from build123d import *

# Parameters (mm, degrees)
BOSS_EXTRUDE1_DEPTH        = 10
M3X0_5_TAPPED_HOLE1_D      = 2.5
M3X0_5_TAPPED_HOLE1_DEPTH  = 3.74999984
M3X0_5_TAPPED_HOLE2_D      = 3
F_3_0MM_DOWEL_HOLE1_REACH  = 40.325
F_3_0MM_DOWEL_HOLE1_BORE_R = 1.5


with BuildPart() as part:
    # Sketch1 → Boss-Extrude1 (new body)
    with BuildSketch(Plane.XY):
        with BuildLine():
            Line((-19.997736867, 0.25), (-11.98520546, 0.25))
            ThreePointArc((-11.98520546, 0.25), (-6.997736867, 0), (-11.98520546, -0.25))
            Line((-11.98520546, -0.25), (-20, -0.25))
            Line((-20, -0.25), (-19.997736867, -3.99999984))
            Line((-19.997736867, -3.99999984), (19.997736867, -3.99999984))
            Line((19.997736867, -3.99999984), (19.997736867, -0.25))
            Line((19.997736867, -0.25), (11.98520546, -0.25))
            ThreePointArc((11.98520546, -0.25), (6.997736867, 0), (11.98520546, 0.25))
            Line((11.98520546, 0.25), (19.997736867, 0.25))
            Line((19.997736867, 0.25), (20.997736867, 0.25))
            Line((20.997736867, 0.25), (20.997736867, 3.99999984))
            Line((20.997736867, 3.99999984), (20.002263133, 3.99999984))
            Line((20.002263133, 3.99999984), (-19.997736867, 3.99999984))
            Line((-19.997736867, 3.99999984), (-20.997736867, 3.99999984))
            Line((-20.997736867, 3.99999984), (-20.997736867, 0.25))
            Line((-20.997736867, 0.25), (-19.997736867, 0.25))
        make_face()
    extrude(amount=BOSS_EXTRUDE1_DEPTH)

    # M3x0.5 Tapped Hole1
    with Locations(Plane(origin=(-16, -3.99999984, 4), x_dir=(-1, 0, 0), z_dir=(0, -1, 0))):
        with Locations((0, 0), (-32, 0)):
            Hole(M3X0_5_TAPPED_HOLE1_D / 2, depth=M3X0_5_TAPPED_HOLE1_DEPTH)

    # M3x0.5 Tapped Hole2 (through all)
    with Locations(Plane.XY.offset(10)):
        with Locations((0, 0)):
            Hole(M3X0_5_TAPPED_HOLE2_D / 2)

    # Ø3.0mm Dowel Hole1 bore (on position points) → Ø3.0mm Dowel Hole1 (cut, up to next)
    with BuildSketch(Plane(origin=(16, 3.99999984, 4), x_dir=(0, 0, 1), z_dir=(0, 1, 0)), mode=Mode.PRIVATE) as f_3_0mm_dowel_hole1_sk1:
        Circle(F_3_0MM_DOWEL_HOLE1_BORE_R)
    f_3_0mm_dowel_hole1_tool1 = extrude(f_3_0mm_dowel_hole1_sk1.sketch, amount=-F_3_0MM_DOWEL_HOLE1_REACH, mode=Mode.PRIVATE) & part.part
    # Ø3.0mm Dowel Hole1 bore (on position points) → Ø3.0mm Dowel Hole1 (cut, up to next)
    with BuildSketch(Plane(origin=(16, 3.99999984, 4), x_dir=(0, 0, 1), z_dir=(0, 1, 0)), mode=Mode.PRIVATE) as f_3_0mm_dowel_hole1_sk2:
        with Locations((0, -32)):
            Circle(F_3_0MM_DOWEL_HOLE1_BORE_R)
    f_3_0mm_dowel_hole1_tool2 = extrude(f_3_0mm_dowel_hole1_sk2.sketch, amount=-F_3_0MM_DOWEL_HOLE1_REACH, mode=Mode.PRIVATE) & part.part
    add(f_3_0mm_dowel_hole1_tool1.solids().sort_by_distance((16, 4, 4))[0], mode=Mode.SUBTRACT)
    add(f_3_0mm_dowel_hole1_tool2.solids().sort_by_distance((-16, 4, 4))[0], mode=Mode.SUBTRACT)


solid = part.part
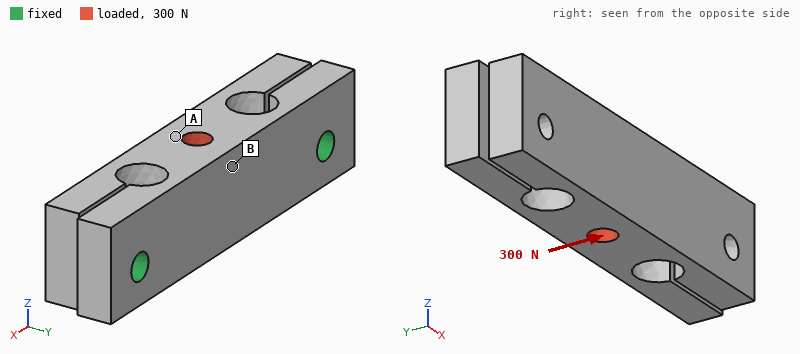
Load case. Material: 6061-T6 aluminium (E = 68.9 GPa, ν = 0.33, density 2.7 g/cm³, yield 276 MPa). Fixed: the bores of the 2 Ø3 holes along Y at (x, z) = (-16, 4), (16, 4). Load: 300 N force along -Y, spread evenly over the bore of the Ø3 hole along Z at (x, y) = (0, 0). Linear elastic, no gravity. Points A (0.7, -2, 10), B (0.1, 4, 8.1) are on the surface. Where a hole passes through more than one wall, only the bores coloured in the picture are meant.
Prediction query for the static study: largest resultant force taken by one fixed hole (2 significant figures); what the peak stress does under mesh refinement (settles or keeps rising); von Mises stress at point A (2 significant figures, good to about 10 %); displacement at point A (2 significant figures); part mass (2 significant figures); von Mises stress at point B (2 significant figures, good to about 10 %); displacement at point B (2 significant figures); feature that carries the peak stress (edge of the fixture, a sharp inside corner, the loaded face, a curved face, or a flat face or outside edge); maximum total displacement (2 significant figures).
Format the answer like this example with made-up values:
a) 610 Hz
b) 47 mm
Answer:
a) 150 N
b) keeps rising
c) 7.1 MPa
d) 14 µm
e) 7.1 g
f) 15 MPa
g) 13 µm
h) edge of the fixture
i) 14 µm
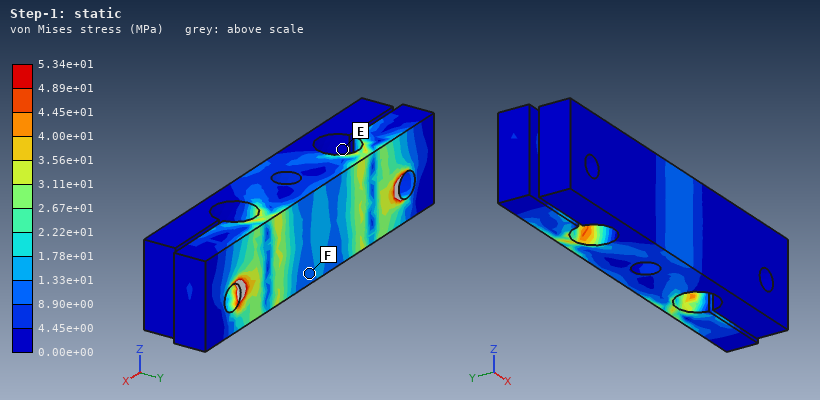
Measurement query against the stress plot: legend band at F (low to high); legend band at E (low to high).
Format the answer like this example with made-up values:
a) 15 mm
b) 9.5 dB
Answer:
a) 8.90e+00 to 1.33e+01 MPa
b) 0.00e+00 to 4.45e+00 MPa
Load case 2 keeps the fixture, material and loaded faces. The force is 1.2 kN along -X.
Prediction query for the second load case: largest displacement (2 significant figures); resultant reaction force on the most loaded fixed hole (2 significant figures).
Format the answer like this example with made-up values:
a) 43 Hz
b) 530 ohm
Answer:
a) 35 µm
b) 630 N
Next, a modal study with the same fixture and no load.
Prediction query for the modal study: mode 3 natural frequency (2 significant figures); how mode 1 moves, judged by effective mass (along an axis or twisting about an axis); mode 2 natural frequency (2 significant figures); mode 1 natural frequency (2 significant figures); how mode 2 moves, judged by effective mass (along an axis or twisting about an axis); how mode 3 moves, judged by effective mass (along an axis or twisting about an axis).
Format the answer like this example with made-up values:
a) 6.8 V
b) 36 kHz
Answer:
a) 6900 Hz
b) twisting about Z
c) 5700 Hz
d) 5400 Hz
e) along Y
f) along Z
